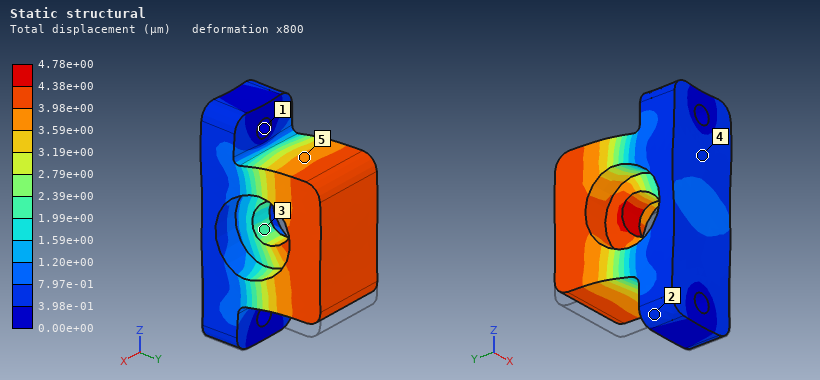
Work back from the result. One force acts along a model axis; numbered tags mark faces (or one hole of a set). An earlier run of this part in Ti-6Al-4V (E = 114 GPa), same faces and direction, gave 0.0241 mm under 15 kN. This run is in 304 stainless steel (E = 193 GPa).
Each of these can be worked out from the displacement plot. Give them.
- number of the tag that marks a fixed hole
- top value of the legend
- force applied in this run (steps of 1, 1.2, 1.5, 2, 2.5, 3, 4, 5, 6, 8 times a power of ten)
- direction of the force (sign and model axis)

1
4.78e+00 µm
5 kN
+Z
